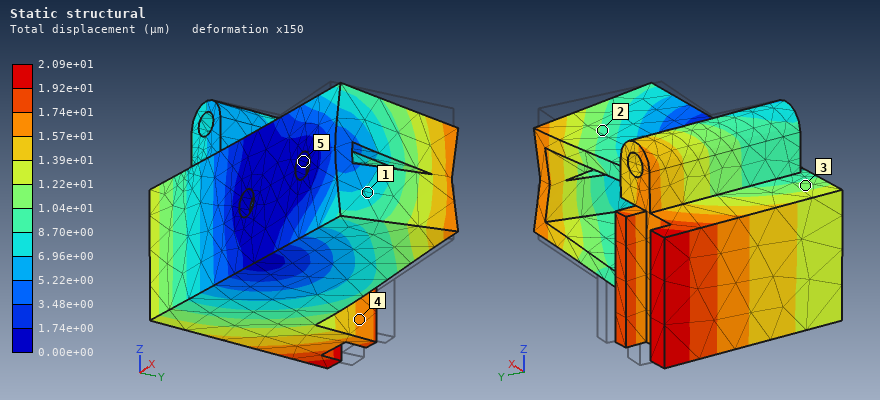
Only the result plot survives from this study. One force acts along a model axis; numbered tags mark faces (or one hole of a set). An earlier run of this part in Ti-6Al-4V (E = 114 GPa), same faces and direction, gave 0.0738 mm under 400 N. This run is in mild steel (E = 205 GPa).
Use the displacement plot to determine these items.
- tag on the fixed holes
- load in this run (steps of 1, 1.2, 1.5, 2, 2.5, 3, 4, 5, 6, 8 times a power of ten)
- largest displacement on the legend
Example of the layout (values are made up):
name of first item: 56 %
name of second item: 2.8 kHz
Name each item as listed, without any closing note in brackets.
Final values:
tag on the fixed holes: 5
load in this run: 200 N
largest displacement on the legend: 2.09e+01 µm
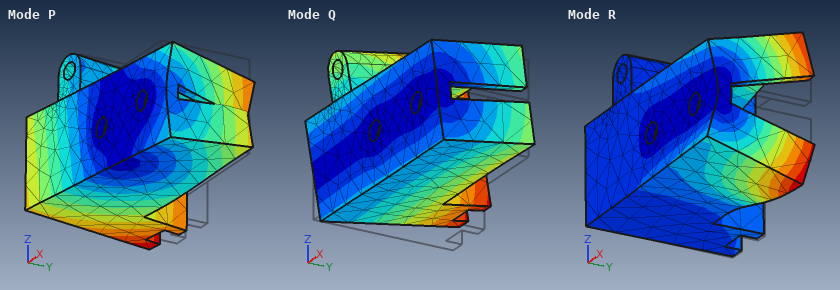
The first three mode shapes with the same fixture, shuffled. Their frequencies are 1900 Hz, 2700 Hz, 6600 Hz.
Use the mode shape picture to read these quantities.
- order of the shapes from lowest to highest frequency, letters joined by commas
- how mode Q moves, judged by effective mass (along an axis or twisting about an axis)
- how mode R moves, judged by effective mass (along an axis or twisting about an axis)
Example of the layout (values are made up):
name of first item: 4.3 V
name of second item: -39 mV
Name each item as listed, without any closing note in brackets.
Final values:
order of the shapes from lowest to highest frequency, letters joined by commas: Q, P, R
how mode Q moves, judged by effective mass: along Z
how mode R moves, judged by effective mass: along Y
